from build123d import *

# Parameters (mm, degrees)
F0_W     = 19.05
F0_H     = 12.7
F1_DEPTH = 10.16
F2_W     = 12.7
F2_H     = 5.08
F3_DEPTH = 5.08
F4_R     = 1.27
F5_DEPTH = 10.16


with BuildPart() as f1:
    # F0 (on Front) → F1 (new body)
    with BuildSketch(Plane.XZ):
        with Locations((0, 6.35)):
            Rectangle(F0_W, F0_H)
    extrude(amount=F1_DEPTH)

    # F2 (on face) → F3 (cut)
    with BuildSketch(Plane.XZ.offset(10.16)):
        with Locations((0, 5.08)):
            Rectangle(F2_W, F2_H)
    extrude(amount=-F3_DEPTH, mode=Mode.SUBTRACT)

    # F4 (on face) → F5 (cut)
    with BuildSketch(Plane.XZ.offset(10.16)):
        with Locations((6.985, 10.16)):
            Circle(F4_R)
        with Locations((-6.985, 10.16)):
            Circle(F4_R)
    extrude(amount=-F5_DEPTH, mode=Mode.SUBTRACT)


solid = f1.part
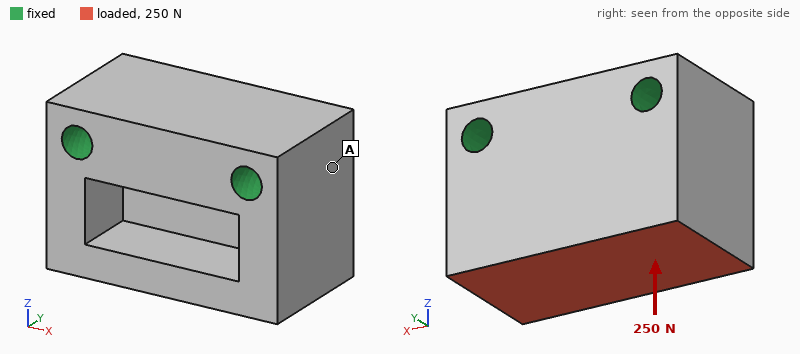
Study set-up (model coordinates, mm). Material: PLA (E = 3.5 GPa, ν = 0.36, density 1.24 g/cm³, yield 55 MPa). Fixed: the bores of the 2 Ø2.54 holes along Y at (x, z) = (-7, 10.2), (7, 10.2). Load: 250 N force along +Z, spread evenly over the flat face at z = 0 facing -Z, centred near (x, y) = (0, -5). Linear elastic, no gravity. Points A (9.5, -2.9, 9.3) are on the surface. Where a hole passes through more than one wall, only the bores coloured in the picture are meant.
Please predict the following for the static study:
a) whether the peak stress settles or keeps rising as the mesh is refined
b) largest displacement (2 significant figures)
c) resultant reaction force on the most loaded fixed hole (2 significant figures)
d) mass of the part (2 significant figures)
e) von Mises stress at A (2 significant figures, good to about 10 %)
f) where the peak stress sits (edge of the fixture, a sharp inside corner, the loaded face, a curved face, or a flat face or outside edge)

keeps rising
42 µm
130 N
2.5 g
1.2 MPa
a sharp inside corner
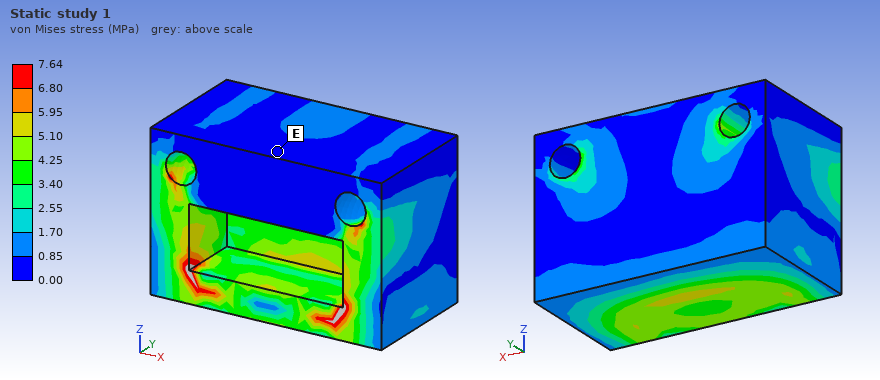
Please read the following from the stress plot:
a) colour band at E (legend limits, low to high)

0.00 to 0.85 MPa
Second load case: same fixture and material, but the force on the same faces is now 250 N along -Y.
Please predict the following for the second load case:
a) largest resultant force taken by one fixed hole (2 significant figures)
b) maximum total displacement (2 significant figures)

130 N
79 µm
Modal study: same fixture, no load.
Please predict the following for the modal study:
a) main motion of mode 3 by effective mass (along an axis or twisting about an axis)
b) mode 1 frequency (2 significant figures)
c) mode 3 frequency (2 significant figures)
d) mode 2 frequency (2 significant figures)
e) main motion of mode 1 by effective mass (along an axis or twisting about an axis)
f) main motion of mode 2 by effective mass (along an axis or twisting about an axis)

along X
13 kHz
21 kHz
16 kHz
along Y
along X
